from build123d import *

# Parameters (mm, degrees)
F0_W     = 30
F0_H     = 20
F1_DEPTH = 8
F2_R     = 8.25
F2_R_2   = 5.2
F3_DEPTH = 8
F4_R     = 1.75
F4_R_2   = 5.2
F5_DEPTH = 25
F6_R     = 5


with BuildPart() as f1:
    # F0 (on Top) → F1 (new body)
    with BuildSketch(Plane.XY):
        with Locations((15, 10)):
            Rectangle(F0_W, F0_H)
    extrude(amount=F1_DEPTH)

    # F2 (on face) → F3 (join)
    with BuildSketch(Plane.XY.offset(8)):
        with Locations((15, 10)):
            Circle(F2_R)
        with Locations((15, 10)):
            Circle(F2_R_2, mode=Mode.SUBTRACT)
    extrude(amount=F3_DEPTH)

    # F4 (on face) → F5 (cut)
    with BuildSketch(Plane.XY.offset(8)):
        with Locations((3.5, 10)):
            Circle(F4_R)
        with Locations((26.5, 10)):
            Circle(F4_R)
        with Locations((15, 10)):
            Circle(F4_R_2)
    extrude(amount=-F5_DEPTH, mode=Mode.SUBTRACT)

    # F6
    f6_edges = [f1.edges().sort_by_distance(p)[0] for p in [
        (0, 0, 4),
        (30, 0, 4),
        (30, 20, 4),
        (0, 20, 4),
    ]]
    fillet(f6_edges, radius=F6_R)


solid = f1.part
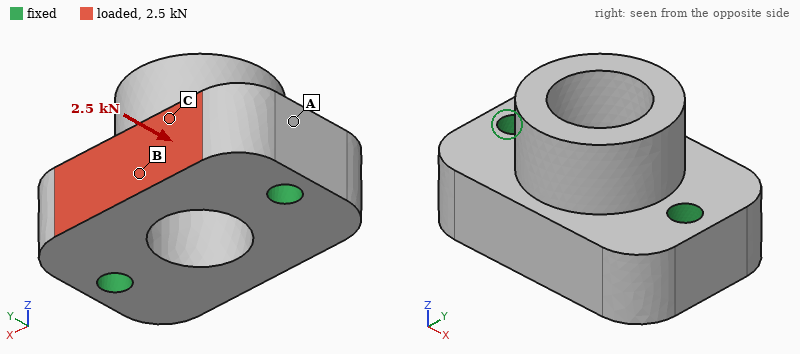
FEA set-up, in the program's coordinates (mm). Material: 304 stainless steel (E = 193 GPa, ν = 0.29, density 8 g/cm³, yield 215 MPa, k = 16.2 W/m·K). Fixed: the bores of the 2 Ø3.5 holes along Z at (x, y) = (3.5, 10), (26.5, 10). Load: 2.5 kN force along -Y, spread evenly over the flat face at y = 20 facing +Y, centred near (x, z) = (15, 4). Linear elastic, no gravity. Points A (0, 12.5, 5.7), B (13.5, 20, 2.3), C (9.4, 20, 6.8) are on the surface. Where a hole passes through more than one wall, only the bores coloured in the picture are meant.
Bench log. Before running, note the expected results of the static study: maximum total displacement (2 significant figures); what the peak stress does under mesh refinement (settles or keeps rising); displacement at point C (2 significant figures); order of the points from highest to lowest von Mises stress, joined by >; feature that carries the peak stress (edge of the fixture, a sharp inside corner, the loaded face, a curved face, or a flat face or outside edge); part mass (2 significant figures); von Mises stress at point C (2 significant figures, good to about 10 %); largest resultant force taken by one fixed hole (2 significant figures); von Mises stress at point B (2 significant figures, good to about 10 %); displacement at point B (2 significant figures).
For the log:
2.5 µm
keeps rising
1.5 µm
B > C > A
edge of the fixture
39 g
15 MPa
1.3 kN
27 MPa
2.3 µm
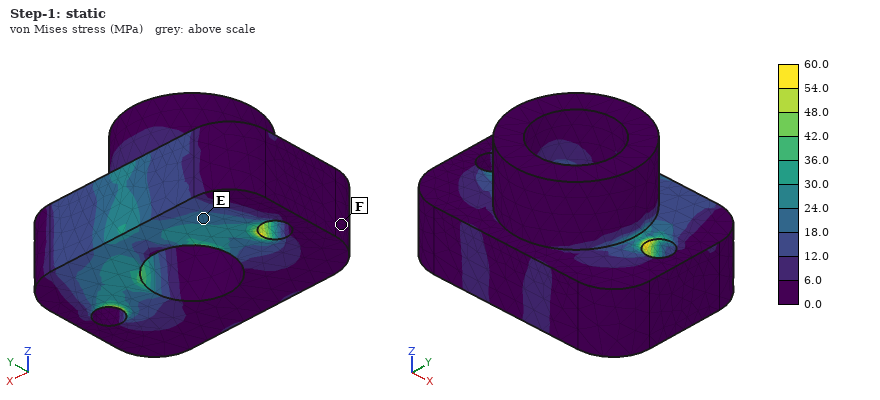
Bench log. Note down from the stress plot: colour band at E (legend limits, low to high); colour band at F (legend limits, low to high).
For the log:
18.0 to 24.0 MPa
0.0 to 6.0 MPa
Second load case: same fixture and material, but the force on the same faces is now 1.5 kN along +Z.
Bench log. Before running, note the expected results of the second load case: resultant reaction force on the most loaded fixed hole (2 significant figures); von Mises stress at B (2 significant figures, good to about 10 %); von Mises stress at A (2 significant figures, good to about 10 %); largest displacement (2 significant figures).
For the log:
760 N
20 MPa
12 MPa
6.5 µm
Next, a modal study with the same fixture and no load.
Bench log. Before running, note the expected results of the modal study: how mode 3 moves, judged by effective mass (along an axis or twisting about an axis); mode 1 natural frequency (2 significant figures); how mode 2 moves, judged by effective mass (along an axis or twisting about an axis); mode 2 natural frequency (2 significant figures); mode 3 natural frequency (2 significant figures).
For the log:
along X
25 kHz
along Z
35 kHz
44 kHz
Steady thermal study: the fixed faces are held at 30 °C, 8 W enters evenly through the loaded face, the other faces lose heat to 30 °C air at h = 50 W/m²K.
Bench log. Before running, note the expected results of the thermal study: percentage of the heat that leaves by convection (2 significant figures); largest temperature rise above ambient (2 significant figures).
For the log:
12 %
34 K
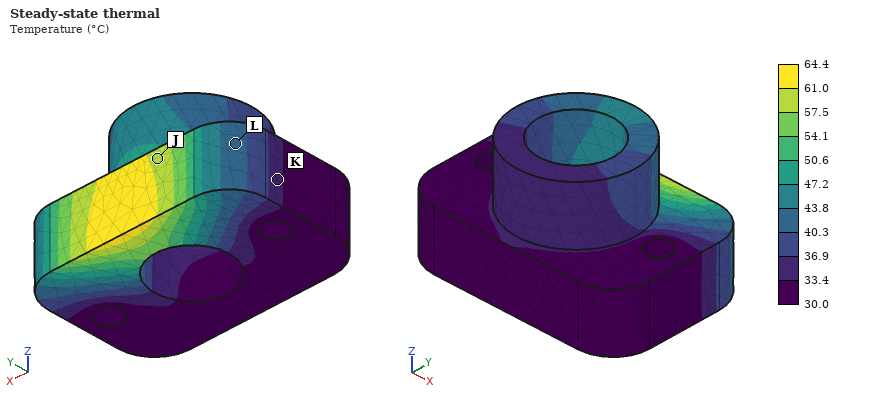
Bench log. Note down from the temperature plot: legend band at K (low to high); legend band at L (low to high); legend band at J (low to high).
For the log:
33.4 to 36.9 °C
40.3 to 43.8 °C
57.5 to 61.0 °C
